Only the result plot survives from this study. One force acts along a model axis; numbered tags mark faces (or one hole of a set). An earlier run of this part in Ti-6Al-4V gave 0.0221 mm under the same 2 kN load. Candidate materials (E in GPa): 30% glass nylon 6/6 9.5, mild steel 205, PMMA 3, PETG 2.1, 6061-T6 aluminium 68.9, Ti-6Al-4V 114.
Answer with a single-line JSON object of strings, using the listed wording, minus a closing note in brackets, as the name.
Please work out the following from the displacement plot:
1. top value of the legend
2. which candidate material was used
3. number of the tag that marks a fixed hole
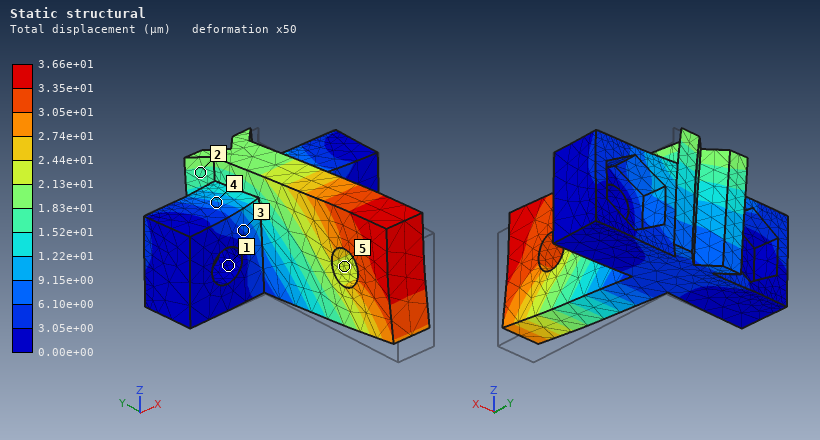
{"top value of the legend": "3.66e+01 µm", "which candidate material was used": "6061-T6 aluminium", "number of the tag that marks a fixed hole": "1"}
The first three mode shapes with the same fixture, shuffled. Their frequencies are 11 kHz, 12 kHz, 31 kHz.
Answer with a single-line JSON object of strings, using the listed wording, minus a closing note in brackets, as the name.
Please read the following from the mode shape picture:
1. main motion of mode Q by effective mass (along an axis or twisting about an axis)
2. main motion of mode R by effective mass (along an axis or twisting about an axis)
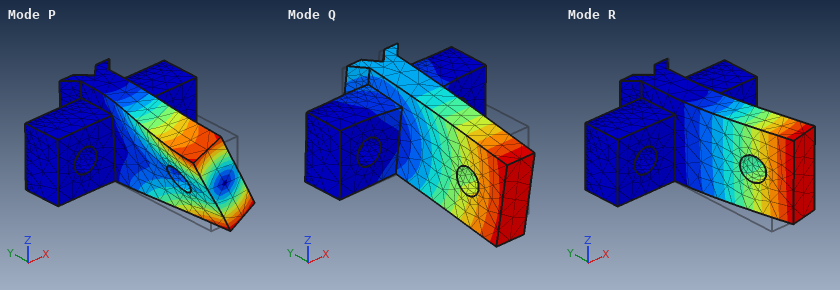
{"main motion of mode Q by effective mass": "along Z", "main motion of mode R by effective mass": "along X"}
